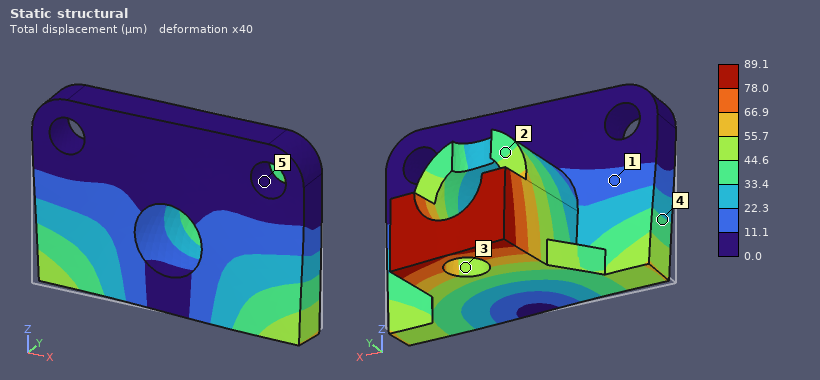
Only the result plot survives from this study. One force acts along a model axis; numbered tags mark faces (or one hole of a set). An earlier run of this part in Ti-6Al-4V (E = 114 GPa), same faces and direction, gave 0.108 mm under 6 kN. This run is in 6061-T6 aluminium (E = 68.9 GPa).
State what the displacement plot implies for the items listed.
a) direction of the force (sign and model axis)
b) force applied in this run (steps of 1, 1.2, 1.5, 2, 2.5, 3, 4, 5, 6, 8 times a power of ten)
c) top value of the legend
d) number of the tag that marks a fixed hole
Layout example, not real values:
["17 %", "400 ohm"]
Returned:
["+X", "3 kN", "89.1 µm", "5"]
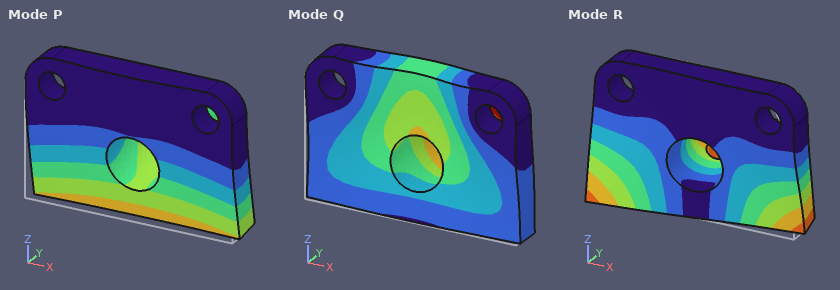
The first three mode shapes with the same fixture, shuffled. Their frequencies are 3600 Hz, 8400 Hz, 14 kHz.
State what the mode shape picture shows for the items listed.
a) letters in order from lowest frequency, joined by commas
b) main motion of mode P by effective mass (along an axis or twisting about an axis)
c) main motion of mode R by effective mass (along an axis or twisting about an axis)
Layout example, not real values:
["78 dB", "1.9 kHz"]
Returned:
["P, R, Q", "along Y", "along X"]
